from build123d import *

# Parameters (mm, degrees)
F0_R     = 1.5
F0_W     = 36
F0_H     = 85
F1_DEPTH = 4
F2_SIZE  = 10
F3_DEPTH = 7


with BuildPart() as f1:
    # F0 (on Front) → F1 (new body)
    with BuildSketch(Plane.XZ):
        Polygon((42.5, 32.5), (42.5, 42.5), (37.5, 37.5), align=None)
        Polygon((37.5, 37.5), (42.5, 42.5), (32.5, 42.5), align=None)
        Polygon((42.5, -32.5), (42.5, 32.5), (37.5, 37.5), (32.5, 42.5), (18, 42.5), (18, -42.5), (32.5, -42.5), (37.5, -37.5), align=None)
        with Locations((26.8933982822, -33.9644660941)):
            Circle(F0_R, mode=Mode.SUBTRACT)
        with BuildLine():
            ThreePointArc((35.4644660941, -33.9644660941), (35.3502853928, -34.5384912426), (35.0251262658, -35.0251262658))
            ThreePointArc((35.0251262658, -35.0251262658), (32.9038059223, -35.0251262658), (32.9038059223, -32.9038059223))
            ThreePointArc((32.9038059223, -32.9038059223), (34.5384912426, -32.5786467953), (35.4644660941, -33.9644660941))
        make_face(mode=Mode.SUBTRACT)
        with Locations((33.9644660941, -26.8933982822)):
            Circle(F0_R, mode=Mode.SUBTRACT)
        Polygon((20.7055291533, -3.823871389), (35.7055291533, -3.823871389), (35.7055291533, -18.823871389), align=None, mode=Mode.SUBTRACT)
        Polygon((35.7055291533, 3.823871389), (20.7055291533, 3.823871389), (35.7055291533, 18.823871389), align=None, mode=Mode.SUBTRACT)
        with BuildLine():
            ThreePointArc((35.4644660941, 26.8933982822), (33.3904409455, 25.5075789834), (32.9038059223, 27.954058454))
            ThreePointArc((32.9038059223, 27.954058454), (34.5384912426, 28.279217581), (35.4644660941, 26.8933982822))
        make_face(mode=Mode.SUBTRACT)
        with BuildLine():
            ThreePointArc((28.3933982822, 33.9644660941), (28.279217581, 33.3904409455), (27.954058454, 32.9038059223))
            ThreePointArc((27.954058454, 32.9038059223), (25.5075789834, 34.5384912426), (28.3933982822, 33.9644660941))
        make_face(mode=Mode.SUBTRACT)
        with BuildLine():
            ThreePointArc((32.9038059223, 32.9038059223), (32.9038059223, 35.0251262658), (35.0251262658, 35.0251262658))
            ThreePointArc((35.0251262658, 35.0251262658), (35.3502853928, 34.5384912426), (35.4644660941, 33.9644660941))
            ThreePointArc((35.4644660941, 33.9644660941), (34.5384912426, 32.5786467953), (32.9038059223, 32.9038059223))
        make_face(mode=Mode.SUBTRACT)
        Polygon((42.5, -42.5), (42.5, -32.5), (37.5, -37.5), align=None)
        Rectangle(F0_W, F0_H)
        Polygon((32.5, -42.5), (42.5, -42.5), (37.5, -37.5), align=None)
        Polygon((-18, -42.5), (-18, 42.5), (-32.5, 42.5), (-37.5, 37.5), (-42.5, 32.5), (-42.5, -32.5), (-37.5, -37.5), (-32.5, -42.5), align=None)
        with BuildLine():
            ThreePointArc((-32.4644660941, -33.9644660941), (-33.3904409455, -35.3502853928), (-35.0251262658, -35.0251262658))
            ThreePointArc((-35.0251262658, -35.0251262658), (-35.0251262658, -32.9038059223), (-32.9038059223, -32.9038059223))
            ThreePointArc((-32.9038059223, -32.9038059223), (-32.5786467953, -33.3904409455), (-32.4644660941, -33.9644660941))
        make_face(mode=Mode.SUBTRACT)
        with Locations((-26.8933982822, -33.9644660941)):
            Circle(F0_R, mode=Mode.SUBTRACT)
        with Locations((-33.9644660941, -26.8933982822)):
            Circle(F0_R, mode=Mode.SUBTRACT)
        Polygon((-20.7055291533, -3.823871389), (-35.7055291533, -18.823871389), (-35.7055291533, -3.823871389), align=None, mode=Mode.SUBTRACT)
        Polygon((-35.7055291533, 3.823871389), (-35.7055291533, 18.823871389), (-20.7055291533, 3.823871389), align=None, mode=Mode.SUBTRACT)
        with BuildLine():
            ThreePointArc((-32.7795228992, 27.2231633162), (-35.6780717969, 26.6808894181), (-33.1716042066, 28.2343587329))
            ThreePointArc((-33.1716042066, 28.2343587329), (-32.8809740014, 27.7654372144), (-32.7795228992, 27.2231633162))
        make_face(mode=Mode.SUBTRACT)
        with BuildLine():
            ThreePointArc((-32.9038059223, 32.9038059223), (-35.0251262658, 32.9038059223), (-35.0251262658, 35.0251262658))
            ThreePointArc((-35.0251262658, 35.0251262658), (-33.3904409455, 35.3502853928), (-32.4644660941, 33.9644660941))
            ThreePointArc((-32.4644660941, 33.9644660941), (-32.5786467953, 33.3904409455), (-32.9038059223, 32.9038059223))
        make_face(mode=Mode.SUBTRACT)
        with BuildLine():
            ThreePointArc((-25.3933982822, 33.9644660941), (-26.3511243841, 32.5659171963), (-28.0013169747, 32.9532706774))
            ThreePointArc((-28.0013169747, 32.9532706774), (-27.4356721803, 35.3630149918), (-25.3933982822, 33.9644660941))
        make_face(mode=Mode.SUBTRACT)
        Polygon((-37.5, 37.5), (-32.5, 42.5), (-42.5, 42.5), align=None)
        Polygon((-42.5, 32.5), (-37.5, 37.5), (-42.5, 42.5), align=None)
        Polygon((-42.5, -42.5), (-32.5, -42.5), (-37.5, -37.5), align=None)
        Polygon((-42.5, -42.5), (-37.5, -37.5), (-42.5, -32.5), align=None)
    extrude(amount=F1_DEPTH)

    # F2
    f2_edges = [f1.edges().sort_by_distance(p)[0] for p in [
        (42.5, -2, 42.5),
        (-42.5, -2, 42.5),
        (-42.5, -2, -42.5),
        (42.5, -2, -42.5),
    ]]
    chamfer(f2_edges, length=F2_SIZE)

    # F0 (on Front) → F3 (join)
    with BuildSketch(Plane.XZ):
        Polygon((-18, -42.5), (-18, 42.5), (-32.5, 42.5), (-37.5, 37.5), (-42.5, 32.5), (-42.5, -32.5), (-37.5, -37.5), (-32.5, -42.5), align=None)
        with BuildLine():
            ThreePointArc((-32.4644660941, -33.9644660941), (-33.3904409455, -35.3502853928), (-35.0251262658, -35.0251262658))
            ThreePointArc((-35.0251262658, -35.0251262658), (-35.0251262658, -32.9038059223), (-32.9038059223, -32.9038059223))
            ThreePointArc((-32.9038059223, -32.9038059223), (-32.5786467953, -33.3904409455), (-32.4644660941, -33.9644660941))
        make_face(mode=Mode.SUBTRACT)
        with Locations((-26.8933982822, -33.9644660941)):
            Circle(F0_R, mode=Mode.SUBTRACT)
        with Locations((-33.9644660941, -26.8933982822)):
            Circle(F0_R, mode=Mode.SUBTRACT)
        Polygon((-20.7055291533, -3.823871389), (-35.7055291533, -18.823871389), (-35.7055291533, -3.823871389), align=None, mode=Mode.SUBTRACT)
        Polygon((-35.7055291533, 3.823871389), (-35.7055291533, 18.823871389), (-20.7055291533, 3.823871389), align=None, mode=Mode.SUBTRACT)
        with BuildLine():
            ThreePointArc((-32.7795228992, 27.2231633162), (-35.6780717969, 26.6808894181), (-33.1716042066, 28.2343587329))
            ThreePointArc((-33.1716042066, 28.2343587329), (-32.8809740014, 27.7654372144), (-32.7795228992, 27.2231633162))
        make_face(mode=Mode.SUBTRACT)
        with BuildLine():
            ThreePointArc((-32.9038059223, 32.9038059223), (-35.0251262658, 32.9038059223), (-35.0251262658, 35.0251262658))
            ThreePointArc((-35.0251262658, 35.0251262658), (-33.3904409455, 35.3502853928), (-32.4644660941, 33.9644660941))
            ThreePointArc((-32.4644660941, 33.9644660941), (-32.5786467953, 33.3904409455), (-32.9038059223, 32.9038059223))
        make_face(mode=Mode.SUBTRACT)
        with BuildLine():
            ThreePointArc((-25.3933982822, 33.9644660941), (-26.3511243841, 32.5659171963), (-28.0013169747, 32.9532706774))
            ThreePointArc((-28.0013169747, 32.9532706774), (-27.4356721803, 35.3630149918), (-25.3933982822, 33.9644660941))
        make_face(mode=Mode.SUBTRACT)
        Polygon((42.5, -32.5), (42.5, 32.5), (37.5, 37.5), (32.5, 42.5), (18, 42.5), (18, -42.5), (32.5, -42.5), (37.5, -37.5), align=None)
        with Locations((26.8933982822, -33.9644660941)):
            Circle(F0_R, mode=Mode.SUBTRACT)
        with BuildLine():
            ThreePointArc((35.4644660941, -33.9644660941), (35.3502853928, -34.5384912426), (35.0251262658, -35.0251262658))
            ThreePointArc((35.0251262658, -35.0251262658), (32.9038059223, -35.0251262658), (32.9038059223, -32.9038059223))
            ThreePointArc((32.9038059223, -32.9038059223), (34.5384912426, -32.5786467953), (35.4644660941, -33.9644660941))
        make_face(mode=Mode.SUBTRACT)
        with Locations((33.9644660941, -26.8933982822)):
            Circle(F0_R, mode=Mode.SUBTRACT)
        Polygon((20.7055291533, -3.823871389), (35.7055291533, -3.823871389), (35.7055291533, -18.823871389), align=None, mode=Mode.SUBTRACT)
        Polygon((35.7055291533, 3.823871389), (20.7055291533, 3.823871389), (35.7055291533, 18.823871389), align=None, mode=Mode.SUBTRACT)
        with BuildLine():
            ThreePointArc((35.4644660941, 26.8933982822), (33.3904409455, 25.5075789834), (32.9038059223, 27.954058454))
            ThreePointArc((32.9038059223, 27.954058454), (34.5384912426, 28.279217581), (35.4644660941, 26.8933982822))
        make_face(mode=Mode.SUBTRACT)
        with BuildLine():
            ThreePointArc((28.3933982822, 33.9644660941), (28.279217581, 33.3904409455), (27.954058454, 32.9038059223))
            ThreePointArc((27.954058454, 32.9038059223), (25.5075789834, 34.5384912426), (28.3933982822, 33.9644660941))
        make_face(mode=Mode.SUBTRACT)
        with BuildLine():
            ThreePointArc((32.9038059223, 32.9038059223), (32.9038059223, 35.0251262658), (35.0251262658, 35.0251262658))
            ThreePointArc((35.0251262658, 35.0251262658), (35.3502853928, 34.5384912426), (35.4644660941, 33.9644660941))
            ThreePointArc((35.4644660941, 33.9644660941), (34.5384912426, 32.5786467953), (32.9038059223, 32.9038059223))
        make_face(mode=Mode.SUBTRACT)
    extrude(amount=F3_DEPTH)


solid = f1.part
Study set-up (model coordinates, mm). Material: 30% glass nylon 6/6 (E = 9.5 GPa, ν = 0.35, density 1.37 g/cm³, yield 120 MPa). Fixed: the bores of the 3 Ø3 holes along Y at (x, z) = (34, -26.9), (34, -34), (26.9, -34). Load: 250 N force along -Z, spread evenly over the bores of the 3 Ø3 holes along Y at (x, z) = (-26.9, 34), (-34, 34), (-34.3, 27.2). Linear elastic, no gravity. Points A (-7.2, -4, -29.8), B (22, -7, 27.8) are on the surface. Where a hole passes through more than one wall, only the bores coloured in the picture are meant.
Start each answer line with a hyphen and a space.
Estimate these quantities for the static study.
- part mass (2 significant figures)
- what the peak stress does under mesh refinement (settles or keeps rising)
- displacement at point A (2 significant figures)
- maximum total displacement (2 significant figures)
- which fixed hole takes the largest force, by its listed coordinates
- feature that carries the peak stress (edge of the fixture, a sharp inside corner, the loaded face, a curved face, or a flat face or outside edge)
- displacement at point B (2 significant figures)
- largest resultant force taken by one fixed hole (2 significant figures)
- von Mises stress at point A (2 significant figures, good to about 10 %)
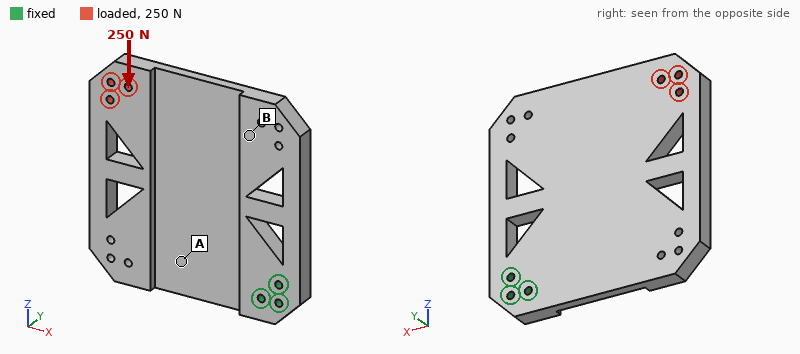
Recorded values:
- 50 g
- keeps rising
- 0.13 mm
- 0.44 mm
- (26.9, -34)
- edge of the fixture
- 0.22 mm
- 1.1 kN
- 4.1 MPa
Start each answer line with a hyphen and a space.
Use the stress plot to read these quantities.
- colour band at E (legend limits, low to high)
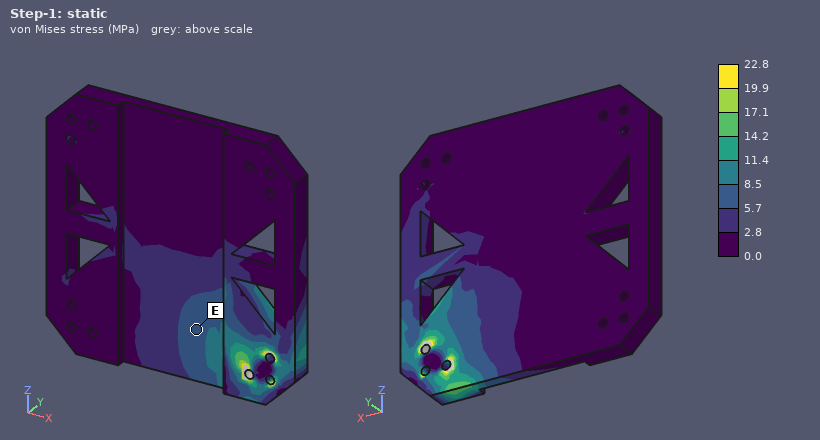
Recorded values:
- 5.7 to 8.5 MPa
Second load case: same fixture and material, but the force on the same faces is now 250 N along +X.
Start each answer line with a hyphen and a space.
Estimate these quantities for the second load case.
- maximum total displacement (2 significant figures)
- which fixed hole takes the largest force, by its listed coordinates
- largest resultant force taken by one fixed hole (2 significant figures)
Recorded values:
- 0.37 mm
- (34, -26.9)
- 1.1 kN
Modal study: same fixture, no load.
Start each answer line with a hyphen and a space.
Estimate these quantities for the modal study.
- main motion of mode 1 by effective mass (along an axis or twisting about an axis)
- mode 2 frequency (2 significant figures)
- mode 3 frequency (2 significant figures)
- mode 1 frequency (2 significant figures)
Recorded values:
- along Y
- 460 Hz
- 860 Hz
- 240 Hz
